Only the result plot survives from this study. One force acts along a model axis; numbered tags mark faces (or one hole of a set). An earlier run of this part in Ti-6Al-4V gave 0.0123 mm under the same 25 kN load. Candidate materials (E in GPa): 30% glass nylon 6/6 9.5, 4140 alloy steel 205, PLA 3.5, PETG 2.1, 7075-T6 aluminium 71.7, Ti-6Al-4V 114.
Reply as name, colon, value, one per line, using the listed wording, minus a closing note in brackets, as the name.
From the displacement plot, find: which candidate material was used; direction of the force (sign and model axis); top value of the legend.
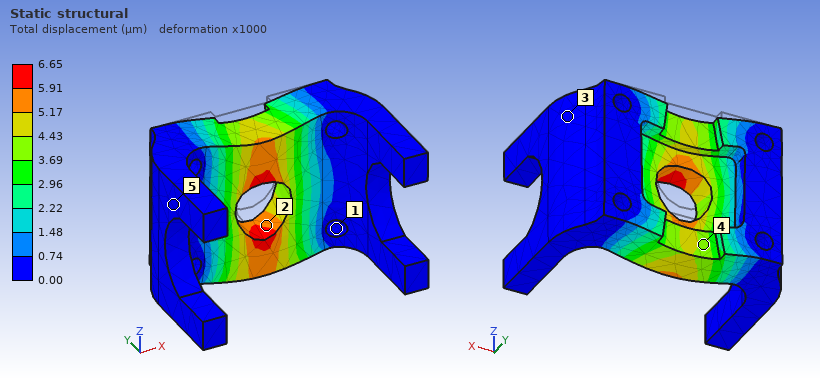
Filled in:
which candidate material was used: 4140 alloy steel
direction of the force: -Z
top value of the legend: 6.65 µm
